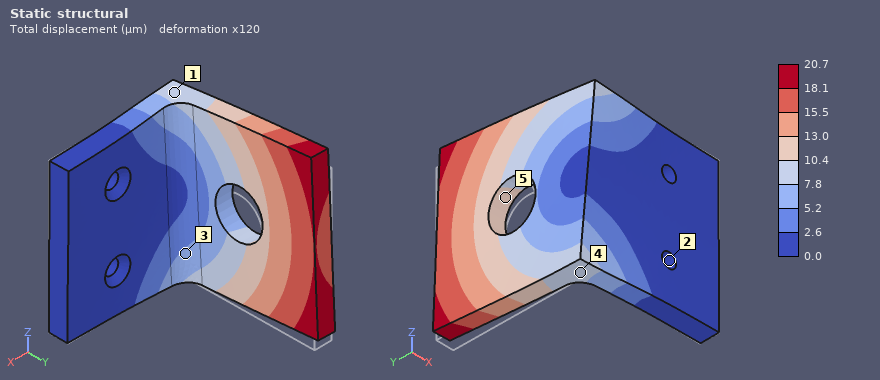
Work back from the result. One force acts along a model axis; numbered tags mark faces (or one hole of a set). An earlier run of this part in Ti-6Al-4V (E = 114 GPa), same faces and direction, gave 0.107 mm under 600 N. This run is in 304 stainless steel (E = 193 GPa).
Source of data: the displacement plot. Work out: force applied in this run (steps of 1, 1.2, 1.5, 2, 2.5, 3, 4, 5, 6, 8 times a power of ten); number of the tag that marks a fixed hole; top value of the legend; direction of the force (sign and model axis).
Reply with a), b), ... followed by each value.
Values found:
a) 200 N
b) 2
c) 20.7 µm
d) +Z
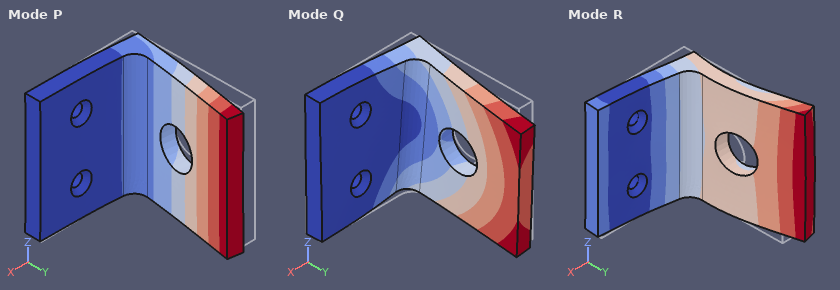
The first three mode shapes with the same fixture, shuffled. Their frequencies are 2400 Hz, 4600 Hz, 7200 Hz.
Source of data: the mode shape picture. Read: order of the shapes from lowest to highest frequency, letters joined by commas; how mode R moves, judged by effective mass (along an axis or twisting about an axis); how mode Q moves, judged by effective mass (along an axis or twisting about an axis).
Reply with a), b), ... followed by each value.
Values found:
a) P, Q, R
b) along Y
c) along Z
